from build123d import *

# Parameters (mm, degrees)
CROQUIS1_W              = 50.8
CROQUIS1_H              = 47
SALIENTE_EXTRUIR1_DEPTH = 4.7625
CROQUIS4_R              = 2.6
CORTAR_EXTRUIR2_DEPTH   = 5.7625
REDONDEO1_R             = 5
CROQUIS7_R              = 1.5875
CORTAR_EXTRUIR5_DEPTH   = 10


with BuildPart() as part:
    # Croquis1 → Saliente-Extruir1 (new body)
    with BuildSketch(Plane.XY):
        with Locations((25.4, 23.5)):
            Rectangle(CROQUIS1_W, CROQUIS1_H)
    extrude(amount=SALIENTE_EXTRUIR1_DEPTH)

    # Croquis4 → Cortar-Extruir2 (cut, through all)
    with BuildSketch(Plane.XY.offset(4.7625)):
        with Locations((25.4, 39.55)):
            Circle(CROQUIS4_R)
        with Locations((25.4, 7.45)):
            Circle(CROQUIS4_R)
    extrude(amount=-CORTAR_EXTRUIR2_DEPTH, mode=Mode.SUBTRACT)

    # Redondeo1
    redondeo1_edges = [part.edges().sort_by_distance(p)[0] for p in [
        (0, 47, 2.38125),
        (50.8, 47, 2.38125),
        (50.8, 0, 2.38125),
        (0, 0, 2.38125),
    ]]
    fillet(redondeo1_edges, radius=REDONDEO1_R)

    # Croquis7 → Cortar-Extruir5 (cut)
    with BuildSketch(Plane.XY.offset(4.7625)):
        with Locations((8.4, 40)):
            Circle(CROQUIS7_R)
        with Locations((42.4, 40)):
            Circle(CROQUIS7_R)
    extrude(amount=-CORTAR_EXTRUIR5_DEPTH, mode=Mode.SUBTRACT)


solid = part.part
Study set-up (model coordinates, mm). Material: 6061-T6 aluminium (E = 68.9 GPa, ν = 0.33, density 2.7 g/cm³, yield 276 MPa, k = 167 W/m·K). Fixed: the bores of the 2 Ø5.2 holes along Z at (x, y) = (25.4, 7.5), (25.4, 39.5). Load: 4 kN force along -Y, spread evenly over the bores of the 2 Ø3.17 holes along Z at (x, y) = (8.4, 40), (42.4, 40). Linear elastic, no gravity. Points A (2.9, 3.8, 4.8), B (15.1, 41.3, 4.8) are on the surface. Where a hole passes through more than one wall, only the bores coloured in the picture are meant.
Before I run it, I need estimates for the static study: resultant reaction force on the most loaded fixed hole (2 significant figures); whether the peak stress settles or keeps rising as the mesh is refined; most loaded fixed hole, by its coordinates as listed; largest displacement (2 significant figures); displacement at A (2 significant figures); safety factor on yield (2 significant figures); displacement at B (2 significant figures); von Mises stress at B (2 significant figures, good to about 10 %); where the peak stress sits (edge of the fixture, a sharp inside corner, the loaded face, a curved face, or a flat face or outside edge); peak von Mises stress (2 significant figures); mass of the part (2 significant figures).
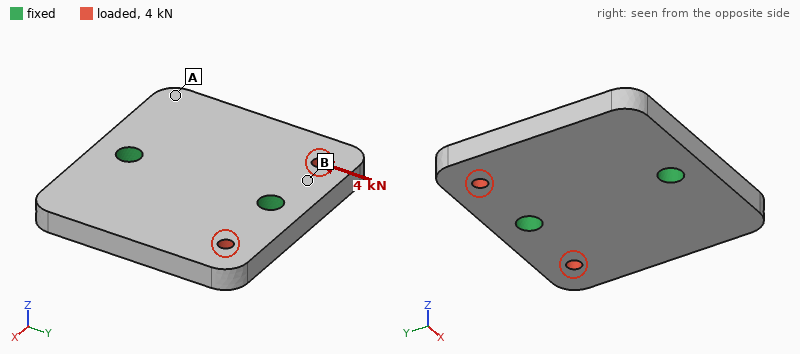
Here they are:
2.2 kN
settles
(25.4, 39.5)
14 µm
7.2 µm
3.2
6.7 µm
21 MPa
the loaded face
87 MPa
30 g
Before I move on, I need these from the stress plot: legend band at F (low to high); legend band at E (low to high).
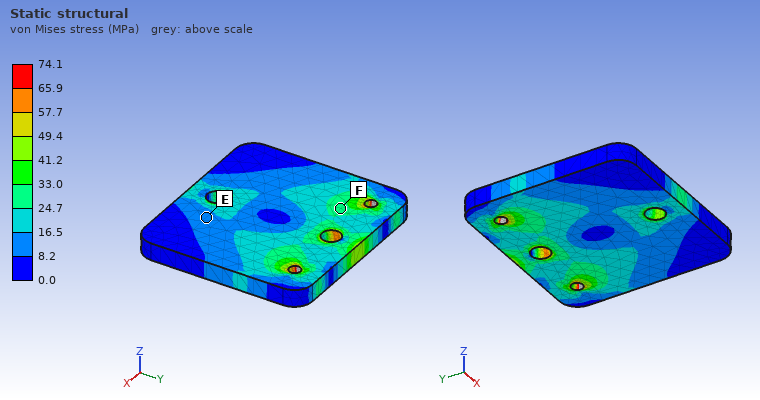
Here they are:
24.7 to 33.0 MPa
8.2 to 16.5 MPa
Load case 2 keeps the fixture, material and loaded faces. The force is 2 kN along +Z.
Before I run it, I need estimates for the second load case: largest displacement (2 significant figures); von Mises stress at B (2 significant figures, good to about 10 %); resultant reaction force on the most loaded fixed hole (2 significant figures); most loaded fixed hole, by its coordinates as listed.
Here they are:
0.15 mm
66 MPa
2.0 kN
(25.4, 39.5)
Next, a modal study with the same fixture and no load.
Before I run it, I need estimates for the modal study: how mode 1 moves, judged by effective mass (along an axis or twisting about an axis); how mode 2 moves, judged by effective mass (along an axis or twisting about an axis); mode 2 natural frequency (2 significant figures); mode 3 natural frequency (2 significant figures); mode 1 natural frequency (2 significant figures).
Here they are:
twisting about Y
along Z
6500 Hz
9900 Hz
5400 Hz
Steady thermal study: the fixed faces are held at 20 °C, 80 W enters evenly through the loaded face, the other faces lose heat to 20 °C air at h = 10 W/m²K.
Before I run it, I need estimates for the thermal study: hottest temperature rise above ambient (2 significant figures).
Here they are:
46 K
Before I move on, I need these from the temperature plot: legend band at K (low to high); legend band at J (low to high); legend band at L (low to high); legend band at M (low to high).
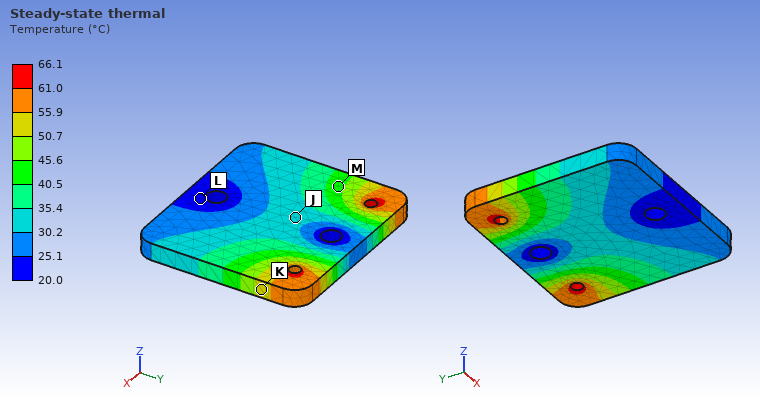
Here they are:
50.7 to 55.9 °C
30.2 to 35.4 °C
20.0 to 25.1 °C
40.5 to 45.6 °C
